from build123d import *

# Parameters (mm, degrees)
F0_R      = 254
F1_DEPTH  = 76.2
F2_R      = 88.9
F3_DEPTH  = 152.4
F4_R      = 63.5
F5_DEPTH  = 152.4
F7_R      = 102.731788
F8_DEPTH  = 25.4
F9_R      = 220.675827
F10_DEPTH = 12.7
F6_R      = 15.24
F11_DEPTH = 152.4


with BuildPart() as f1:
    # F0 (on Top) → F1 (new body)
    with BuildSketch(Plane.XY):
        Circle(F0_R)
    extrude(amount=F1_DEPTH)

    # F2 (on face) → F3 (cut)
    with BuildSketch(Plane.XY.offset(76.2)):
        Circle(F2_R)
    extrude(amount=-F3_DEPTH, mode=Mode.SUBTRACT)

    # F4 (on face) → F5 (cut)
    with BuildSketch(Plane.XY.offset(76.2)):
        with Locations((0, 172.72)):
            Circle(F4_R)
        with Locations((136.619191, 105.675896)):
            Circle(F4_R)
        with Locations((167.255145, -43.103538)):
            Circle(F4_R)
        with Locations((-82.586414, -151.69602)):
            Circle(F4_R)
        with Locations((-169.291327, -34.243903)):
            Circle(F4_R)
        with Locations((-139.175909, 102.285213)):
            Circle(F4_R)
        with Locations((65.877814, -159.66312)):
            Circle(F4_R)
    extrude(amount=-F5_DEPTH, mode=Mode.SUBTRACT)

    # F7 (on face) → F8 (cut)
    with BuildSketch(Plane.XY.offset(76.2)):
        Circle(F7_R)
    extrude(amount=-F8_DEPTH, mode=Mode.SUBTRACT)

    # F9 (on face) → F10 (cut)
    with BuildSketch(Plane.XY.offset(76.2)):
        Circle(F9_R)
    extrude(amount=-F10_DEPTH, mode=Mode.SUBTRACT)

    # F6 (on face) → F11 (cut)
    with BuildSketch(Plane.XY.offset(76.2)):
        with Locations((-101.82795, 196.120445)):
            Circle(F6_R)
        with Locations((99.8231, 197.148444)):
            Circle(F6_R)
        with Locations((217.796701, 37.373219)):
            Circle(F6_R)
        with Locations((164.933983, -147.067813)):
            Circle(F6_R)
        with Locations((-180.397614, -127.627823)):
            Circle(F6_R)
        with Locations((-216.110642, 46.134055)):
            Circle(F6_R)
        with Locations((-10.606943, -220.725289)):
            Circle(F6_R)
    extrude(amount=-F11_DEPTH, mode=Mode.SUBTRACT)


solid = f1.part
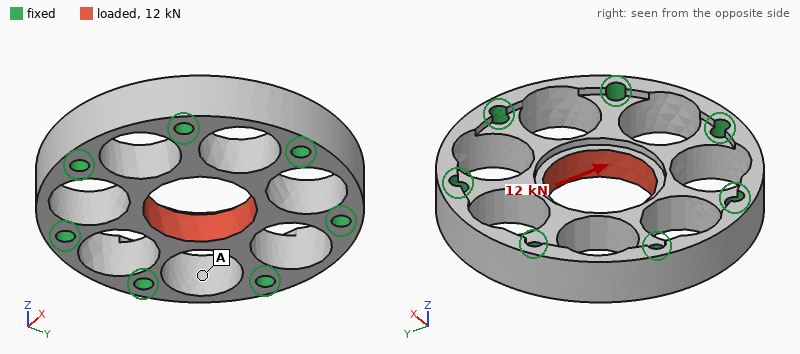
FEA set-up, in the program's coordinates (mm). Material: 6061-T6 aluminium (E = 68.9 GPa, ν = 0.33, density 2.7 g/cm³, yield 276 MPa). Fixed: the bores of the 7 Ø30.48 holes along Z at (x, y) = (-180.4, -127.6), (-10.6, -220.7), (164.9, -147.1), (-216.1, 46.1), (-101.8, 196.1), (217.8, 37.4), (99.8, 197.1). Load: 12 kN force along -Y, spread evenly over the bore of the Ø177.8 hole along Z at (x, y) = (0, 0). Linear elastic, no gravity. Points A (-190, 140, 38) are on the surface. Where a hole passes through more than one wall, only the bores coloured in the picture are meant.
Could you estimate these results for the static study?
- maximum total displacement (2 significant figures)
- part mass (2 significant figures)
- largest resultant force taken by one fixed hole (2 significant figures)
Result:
3.8 µm
15 kg
3.0 kN
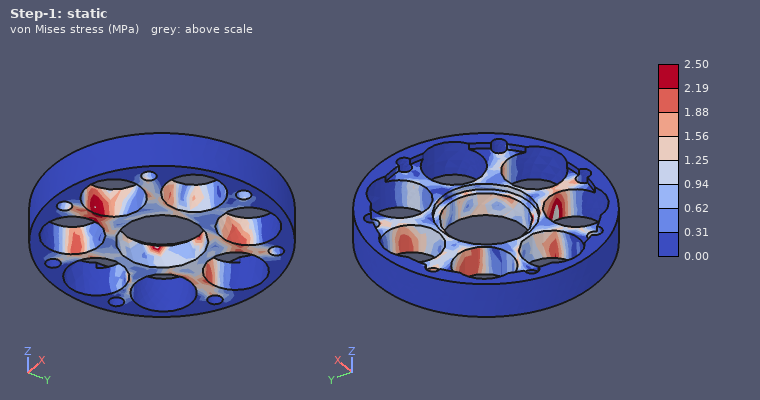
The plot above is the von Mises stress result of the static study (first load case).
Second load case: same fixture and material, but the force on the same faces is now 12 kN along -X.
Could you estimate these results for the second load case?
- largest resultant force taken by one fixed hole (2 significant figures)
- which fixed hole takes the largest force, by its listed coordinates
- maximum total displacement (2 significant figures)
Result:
3.0 kN
(217.8, 37.4)
4.0 µm
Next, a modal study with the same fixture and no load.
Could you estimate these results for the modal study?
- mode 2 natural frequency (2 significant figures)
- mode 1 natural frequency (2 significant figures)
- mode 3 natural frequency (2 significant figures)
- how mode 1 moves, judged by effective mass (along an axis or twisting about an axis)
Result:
3300 Hz
2500 Hz
3300 Hz
along Z
